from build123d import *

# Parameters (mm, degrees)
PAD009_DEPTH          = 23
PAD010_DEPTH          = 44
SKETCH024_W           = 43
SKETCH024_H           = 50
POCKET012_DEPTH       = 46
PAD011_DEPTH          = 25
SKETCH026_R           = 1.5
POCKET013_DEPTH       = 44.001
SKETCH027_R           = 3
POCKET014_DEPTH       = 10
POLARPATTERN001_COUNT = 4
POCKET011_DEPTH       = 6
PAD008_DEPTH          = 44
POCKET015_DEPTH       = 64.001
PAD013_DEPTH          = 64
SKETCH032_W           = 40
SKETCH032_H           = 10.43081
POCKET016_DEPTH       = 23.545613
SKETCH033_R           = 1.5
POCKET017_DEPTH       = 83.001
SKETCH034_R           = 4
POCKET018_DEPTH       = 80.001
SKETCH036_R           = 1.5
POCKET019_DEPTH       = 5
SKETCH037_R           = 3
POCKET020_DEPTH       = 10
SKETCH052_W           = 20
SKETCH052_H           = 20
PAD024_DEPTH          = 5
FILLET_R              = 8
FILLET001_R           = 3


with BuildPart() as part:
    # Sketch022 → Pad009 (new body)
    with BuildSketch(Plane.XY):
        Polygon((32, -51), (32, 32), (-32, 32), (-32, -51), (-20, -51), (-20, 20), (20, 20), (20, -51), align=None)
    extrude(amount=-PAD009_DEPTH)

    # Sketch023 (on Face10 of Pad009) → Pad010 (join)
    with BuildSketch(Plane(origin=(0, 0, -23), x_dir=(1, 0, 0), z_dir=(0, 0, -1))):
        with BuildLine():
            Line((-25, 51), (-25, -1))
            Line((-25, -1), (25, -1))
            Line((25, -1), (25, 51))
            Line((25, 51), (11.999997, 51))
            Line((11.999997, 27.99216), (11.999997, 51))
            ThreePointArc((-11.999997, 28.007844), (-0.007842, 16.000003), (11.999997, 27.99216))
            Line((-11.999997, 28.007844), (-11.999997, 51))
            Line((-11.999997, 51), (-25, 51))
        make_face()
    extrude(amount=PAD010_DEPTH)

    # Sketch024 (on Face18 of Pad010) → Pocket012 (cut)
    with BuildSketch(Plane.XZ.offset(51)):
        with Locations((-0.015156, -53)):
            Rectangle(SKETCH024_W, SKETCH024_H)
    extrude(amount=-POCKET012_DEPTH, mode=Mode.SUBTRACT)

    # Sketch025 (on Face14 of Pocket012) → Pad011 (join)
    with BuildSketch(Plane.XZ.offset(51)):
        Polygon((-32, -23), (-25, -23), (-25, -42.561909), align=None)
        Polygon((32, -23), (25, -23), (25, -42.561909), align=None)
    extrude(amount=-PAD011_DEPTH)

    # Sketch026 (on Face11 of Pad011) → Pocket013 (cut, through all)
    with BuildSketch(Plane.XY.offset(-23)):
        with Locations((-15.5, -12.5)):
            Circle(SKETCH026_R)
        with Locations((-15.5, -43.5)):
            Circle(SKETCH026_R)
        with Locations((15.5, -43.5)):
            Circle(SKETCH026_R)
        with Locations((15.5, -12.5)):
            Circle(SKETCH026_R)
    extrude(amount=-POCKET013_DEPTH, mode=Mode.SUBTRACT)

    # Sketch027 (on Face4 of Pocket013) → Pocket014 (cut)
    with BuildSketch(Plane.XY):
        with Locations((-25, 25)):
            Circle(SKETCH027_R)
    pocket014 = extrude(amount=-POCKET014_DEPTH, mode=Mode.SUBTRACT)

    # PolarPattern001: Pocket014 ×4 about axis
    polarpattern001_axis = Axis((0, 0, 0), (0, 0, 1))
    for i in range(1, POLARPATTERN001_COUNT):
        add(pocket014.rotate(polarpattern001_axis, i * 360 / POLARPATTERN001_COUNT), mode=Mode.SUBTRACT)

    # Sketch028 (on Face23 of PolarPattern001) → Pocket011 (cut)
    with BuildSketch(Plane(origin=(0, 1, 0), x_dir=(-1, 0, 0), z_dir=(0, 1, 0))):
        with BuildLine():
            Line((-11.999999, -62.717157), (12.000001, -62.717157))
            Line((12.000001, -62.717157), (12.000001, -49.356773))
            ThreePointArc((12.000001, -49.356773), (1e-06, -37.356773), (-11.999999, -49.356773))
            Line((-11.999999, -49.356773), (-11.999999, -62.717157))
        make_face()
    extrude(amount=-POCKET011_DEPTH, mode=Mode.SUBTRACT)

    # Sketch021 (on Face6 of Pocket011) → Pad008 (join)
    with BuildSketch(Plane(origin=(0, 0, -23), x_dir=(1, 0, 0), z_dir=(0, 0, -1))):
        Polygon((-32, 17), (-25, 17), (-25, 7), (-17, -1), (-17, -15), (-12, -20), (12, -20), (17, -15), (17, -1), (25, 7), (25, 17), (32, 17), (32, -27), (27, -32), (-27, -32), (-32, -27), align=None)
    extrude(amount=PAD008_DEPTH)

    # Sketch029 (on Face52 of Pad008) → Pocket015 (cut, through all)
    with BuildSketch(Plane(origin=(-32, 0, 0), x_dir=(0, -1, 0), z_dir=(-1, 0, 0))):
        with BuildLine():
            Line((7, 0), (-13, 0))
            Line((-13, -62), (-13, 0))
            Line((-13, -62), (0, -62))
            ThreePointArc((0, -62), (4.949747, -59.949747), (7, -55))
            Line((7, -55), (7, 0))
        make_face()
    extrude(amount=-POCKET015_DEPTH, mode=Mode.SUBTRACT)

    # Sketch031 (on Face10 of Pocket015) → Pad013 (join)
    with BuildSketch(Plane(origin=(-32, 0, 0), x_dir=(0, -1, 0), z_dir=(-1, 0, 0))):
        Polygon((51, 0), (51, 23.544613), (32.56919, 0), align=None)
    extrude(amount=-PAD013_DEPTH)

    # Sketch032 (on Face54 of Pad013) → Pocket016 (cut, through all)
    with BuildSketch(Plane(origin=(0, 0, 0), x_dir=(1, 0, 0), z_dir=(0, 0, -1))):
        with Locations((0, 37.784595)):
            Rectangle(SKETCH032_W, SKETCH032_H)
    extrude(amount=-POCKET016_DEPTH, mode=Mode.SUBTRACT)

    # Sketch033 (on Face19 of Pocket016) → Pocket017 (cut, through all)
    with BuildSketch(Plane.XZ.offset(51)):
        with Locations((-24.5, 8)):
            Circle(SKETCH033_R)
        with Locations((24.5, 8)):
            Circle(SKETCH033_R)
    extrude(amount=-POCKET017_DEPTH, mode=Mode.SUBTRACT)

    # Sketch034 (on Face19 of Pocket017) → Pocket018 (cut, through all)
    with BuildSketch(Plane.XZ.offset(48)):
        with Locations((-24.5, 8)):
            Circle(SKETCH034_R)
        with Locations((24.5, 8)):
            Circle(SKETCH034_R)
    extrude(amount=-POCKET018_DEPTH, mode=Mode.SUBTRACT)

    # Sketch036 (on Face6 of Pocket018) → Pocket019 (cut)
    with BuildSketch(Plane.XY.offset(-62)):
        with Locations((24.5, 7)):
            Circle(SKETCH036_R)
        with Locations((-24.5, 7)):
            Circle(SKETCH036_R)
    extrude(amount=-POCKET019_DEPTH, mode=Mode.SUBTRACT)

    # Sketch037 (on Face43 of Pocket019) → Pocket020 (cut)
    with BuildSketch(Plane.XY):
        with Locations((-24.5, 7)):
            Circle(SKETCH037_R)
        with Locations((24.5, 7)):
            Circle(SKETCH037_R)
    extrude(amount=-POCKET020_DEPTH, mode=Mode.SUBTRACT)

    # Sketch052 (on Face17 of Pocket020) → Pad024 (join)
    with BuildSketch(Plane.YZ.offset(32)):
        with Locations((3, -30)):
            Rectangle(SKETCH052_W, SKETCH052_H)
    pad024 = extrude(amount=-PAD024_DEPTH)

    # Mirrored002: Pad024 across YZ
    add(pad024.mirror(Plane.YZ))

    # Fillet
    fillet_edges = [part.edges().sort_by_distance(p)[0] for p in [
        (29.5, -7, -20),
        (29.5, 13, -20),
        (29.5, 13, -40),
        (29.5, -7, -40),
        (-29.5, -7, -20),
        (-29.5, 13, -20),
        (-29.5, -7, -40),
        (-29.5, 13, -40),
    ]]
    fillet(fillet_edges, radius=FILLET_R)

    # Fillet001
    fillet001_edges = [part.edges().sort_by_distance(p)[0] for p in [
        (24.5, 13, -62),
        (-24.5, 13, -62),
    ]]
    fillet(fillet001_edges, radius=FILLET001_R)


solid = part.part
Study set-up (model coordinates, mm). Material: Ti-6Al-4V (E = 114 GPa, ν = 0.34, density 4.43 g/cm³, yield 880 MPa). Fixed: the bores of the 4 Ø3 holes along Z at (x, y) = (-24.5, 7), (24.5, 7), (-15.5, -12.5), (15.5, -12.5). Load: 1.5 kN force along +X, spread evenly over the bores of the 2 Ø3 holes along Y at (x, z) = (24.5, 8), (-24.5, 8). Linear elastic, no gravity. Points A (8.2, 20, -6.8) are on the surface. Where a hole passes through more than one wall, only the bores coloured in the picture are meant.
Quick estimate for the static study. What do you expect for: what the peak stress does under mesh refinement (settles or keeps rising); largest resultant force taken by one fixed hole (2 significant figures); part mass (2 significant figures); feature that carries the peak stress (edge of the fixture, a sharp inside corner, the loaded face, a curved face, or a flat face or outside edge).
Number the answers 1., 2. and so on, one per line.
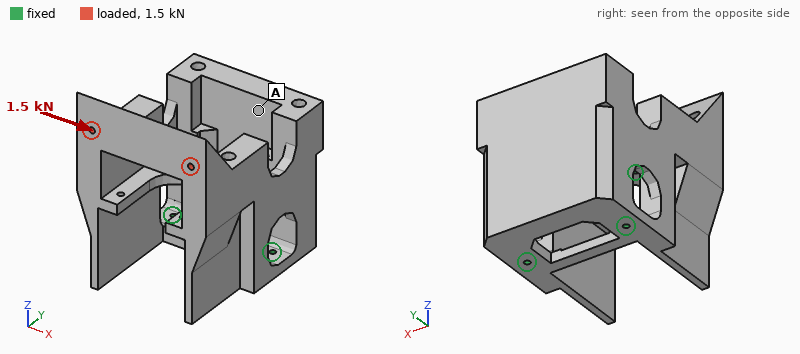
1. keeps rising
2. 1.2 kN
3. 600 g
4. edge of the fixture
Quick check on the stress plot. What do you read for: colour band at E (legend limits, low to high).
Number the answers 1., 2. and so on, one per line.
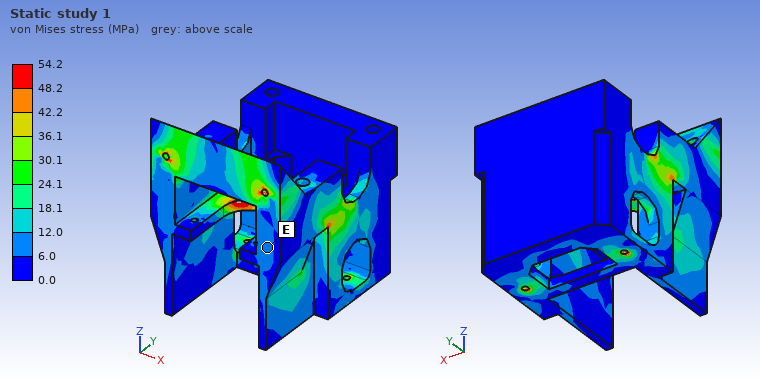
1. 6.0 to 12.0 MPa
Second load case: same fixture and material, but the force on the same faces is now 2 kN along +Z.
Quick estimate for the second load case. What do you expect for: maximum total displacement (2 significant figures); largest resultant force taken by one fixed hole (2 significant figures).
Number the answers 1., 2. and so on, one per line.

1. 48 µm
2. 1.2 kN
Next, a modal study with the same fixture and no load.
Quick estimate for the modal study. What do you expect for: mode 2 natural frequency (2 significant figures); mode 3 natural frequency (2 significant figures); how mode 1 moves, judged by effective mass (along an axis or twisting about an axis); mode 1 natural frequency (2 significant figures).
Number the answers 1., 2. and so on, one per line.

1. 2800 Hz
2. 2900 Hz
3. along Y
4. 2400 Hz
